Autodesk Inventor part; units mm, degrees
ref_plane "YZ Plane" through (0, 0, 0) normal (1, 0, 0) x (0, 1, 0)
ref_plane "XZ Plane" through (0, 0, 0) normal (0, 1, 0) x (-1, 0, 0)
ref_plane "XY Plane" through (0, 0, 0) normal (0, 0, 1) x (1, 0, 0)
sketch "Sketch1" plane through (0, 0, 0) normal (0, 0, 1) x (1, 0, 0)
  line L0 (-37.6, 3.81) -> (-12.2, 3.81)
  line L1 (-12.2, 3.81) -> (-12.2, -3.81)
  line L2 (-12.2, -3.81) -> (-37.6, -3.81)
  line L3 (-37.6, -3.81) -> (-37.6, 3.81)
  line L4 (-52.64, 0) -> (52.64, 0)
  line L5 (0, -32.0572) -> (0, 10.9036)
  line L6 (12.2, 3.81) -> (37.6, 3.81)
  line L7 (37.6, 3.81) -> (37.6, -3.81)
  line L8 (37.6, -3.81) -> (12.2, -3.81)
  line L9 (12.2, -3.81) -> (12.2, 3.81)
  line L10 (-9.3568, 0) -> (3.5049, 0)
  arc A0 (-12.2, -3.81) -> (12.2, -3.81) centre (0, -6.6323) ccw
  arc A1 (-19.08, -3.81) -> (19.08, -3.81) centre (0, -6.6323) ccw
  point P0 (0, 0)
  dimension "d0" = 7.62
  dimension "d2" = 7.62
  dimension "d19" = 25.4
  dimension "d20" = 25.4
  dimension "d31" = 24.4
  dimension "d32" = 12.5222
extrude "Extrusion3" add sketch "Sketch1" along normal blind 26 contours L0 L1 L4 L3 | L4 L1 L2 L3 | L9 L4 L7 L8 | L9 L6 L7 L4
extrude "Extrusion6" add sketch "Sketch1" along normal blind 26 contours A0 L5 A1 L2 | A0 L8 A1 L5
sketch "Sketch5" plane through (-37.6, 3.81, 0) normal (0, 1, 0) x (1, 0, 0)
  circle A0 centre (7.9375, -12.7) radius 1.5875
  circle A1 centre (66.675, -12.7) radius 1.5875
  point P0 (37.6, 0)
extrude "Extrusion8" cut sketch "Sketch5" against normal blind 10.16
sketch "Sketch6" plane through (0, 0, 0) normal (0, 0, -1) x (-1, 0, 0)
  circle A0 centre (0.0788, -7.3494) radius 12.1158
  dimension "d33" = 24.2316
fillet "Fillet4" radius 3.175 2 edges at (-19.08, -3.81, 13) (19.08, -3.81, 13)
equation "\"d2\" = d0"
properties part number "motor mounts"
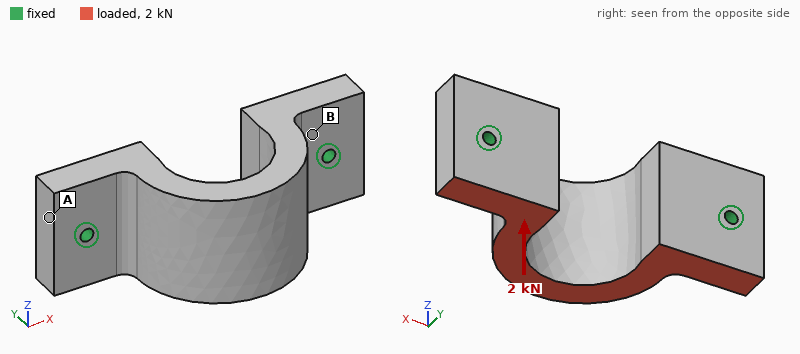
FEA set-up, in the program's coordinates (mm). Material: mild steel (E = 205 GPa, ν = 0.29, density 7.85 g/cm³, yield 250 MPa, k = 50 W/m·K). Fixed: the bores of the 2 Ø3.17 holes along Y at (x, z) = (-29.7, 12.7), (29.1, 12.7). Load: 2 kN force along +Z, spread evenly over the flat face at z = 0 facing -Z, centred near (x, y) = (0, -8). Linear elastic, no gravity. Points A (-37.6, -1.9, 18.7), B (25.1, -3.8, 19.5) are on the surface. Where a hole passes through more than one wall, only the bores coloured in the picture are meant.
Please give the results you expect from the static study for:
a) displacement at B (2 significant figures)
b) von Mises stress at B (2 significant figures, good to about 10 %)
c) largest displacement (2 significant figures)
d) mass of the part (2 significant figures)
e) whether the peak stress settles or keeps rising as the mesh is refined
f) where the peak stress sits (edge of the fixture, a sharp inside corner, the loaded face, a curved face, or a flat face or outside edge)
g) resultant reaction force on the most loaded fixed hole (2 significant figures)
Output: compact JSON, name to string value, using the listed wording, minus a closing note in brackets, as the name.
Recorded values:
{"displacement at B": "3.8 µm", "von Mises stress at B": "25 MPa", "largest displacement": "22 µm", "mass of the part": "160 g", "whether the peak stress settles or keeps rising as the mesh is refined": "keeps rising", "where the peak stress sits": "edge of the fixture", "resultant reaction force on the most loaded fixed hole": "1.0 kN"}
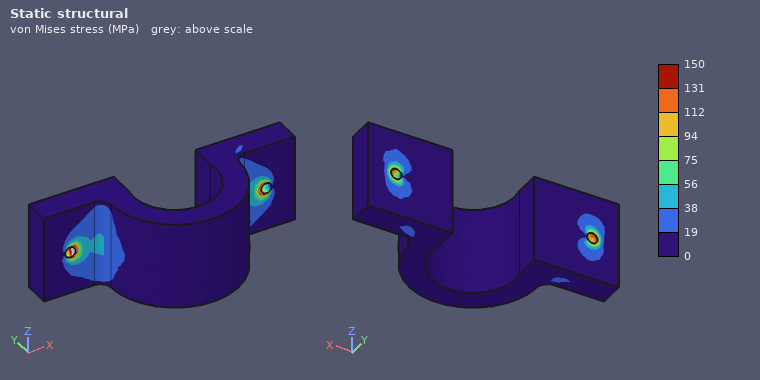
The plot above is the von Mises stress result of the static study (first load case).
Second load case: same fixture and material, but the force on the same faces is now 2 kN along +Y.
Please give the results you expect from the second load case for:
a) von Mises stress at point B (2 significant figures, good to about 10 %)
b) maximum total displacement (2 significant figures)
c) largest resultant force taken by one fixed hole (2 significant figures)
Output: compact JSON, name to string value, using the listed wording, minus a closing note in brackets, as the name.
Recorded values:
{"von Mises stress at point B": "24 MPa", "maximum total displacement": "21 µm", "largest resultant force taken by one fixed hole": "1.1 kN"}
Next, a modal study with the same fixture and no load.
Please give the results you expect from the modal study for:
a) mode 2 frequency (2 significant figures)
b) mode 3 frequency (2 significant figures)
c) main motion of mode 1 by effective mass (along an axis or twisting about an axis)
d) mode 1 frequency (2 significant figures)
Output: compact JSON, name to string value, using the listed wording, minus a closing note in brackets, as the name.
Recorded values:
{"mode 2 frequency": "11 kHz", "mode 3 frequency": "11 kHz", "main motion of mode 1 by effective mass": "along Z", "mode 1 frequency": "4500 Hz"}
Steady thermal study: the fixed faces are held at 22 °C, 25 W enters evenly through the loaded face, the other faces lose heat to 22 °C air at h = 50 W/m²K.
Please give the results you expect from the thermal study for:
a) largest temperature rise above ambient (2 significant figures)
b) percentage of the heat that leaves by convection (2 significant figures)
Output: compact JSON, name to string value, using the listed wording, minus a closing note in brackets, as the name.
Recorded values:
{"largest temperature rise above ambient": "26 K", "percentage of the heat that leaves by convection": "17 %"}
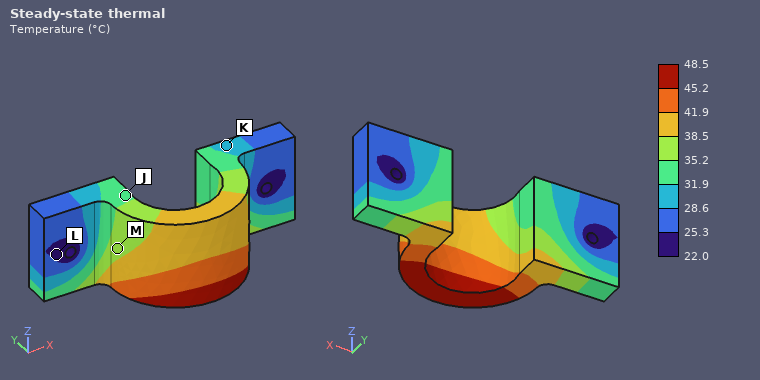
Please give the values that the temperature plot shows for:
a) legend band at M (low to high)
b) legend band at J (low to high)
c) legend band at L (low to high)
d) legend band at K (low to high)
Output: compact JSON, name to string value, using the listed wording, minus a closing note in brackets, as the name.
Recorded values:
{"legend band at M": "35.2 to 38.5 °C", "legend band at J": "31.9 to 35.2 °C", "legend band at L": "22.0 to 25.3 °C", "legend band at K": "28.6 to 31.9 °C"}
